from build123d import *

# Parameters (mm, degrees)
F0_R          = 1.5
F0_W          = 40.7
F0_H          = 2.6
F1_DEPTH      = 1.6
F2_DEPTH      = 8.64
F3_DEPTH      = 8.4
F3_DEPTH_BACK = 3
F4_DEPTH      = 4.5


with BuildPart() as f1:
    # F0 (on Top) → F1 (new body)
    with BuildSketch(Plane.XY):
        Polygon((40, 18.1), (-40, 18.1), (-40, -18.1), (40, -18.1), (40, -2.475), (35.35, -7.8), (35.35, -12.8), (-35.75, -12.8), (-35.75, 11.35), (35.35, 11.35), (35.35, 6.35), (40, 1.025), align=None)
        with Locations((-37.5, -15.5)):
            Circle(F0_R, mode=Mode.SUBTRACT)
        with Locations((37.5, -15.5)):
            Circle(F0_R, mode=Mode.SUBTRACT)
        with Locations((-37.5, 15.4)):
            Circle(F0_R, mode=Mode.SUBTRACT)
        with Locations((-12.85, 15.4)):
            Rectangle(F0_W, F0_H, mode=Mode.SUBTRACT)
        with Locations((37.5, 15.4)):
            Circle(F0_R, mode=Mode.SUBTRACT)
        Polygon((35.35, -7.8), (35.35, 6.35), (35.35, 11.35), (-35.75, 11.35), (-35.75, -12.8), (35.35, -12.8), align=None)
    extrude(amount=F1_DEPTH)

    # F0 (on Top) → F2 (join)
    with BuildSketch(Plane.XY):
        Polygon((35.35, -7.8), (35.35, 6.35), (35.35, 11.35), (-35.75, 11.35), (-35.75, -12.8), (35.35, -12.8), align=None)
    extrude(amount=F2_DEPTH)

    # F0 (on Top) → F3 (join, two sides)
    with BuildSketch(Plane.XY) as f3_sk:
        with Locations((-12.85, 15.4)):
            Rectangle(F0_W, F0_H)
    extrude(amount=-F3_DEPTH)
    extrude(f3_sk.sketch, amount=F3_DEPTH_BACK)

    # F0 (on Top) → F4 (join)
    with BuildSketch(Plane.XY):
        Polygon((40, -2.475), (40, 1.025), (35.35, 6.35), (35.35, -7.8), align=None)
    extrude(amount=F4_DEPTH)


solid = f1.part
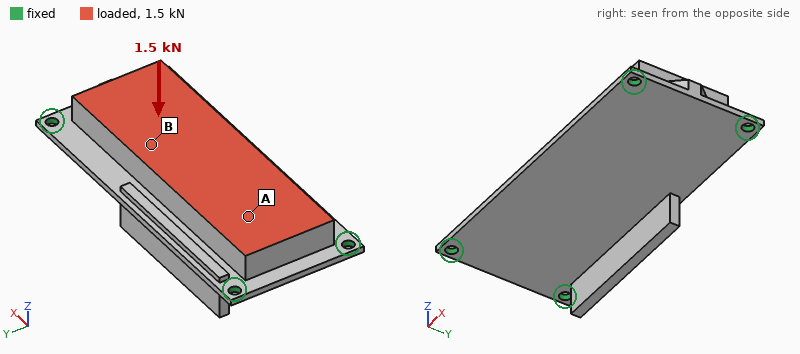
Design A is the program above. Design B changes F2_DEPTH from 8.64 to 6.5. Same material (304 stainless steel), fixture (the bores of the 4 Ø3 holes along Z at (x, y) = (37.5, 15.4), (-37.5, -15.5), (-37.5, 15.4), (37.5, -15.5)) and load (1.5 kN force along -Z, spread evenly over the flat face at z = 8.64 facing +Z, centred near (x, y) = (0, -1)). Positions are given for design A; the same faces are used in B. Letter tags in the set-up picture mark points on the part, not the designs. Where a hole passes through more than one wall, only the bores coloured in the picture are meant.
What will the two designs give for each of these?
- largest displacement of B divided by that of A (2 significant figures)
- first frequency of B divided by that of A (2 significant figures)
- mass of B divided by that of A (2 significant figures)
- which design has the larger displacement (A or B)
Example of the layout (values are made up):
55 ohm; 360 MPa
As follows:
1.7; 0.86; 0.79; B
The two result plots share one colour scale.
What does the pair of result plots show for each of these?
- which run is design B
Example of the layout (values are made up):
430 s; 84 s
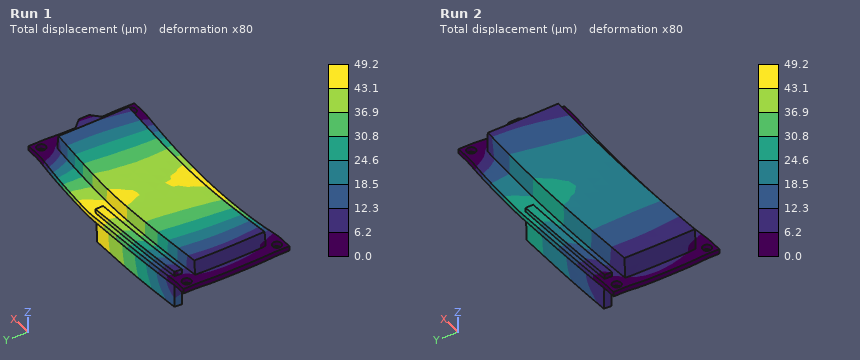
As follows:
Run 1
